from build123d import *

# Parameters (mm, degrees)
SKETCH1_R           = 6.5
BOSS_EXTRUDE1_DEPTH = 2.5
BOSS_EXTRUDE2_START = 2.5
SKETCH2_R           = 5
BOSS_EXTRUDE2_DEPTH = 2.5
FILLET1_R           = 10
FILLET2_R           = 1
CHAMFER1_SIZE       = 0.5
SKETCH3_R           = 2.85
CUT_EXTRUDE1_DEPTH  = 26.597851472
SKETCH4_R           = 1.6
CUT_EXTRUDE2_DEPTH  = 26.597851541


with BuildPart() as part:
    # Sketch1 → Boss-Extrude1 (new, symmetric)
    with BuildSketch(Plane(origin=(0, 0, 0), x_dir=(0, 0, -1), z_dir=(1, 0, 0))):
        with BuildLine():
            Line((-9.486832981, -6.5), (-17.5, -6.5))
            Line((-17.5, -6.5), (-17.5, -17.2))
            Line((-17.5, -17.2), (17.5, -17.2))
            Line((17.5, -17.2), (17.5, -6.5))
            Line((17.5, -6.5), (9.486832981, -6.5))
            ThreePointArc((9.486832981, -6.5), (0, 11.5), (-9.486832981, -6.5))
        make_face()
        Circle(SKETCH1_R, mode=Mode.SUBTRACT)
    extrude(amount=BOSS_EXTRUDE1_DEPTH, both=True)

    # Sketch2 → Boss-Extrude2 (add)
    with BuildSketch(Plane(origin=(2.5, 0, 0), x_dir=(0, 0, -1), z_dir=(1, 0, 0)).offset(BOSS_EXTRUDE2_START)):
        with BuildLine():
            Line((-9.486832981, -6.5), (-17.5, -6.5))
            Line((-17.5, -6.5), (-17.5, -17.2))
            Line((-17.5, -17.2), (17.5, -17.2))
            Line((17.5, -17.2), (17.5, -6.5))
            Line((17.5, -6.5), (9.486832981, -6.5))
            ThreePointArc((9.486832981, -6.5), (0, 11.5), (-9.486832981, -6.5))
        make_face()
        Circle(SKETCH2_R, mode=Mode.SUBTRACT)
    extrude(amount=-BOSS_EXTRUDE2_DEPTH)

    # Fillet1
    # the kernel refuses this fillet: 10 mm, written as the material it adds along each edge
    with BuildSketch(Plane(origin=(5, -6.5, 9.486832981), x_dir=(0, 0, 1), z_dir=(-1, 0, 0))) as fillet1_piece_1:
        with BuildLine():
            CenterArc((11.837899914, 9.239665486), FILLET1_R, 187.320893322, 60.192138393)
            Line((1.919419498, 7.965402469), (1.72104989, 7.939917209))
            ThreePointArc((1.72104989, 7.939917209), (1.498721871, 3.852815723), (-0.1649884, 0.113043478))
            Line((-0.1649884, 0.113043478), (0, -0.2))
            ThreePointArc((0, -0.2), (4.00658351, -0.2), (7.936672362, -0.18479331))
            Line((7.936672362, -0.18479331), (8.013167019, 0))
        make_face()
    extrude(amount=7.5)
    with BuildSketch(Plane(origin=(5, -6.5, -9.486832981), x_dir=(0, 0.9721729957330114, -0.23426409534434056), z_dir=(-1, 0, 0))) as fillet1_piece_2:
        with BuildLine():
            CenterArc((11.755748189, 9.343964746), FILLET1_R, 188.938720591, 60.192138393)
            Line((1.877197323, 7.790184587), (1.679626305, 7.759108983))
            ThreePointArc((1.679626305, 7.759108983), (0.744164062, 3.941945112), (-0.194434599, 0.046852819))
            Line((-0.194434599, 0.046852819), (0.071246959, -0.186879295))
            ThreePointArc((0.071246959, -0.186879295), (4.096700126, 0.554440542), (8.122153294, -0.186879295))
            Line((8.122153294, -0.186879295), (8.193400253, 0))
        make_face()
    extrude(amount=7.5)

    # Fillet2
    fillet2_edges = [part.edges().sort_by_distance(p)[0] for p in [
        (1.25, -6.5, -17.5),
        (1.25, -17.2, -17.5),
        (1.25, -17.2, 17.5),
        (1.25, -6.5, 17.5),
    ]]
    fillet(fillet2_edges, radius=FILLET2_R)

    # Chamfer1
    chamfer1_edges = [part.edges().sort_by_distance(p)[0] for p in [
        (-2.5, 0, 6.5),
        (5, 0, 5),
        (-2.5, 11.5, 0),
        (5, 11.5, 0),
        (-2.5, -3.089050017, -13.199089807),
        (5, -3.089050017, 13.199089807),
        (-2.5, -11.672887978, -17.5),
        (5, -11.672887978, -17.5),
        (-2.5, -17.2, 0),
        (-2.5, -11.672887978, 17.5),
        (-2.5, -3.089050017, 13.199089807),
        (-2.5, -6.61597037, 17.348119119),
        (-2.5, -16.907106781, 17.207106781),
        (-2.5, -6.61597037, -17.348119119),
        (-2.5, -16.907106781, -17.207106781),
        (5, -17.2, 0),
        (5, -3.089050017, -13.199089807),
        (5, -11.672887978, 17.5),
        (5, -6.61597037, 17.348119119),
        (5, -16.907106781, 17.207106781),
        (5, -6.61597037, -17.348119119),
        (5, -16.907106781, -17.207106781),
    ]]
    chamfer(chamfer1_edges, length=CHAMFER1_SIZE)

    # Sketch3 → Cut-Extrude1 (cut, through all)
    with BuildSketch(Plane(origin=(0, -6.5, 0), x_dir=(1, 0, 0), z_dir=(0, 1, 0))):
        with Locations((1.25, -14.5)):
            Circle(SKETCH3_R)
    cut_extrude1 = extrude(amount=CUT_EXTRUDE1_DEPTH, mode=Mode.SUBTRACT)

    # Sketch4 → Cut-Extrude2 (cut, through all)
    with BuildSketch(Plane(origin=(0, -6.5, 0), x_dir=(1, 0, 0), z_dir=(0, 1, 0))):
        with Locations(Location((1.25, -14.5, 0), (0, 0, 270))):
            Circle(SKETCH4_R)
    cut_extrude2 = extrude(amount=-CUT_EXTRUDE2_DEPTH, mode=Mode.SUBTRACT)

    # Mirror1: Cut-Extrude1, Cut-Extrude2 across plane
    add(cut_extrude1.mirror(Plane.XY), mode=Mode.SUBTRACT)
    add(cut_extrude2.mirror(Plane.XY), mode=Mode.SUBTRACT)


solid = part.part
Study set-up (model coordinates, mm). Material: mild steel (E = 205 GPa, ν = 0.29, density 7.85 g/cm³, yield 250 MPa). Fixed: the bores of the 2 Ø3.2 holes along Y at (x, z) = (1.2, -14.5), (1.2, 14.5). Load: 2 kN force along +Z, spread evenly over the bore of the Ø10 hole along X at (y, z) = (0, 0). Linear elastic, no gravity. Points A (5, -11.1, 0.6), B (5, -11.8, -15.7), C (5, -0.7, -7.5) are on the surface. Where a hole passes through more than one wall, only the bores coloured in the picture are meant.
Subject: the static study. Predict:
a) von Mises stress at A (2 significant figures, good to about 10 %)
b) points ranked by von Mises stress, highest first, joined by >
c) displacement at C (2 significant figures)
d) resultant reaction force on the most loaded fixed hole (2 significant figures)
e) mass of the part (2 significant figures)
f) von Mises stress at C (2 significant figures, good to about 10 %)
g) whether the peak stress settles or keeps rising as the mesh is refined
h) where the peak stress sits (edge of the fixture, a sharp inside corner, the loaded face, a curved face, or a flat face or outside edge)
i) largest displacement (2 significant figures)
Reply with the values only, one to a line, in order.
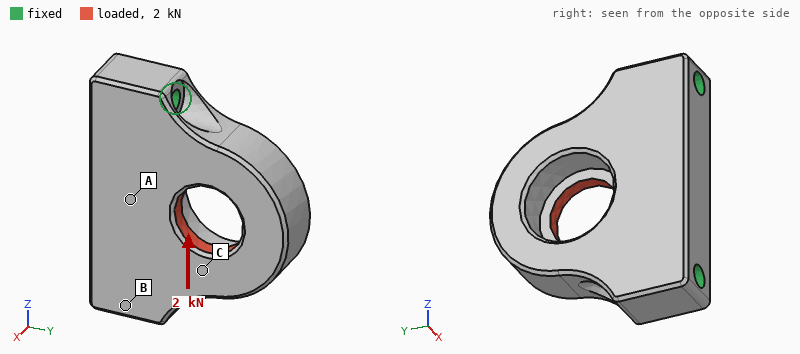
16 MPa
C > A > B
3.3 µm
1.2 kN
35 g
53 MPa
keeps rising
a sharp inside corner
6.3 µm
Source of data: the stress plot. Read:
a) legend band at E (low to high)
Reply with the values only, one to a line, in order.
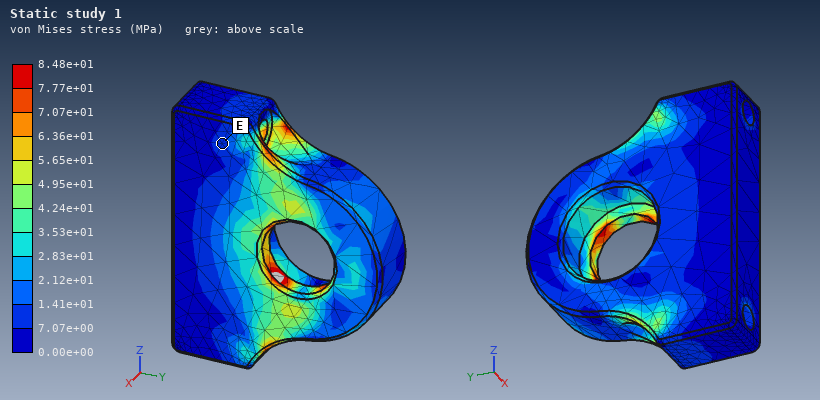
7.07e+00 to 1.41e+01 MPa
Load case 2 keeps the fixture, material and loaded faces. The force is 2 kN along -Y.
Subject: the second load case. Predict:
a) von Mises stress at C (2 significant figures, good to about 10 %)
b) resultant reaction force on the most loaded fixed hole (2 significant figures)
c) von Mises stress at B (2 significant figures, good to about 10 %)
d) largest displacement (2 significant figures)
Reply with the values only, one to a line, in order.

31 MPa
1.0 kN
7.5 MPa
8.7 µm
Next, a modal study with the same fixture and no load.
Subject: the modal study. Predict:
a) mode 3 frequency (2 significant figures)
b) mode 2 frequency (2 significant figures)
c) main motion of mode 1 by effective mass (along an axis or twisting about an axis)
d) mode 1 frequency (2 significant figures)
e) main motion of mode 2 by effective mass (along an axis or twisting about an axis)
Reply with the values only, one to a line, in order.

27 kHz
25 kHz
along X
11 kHz
along Z
